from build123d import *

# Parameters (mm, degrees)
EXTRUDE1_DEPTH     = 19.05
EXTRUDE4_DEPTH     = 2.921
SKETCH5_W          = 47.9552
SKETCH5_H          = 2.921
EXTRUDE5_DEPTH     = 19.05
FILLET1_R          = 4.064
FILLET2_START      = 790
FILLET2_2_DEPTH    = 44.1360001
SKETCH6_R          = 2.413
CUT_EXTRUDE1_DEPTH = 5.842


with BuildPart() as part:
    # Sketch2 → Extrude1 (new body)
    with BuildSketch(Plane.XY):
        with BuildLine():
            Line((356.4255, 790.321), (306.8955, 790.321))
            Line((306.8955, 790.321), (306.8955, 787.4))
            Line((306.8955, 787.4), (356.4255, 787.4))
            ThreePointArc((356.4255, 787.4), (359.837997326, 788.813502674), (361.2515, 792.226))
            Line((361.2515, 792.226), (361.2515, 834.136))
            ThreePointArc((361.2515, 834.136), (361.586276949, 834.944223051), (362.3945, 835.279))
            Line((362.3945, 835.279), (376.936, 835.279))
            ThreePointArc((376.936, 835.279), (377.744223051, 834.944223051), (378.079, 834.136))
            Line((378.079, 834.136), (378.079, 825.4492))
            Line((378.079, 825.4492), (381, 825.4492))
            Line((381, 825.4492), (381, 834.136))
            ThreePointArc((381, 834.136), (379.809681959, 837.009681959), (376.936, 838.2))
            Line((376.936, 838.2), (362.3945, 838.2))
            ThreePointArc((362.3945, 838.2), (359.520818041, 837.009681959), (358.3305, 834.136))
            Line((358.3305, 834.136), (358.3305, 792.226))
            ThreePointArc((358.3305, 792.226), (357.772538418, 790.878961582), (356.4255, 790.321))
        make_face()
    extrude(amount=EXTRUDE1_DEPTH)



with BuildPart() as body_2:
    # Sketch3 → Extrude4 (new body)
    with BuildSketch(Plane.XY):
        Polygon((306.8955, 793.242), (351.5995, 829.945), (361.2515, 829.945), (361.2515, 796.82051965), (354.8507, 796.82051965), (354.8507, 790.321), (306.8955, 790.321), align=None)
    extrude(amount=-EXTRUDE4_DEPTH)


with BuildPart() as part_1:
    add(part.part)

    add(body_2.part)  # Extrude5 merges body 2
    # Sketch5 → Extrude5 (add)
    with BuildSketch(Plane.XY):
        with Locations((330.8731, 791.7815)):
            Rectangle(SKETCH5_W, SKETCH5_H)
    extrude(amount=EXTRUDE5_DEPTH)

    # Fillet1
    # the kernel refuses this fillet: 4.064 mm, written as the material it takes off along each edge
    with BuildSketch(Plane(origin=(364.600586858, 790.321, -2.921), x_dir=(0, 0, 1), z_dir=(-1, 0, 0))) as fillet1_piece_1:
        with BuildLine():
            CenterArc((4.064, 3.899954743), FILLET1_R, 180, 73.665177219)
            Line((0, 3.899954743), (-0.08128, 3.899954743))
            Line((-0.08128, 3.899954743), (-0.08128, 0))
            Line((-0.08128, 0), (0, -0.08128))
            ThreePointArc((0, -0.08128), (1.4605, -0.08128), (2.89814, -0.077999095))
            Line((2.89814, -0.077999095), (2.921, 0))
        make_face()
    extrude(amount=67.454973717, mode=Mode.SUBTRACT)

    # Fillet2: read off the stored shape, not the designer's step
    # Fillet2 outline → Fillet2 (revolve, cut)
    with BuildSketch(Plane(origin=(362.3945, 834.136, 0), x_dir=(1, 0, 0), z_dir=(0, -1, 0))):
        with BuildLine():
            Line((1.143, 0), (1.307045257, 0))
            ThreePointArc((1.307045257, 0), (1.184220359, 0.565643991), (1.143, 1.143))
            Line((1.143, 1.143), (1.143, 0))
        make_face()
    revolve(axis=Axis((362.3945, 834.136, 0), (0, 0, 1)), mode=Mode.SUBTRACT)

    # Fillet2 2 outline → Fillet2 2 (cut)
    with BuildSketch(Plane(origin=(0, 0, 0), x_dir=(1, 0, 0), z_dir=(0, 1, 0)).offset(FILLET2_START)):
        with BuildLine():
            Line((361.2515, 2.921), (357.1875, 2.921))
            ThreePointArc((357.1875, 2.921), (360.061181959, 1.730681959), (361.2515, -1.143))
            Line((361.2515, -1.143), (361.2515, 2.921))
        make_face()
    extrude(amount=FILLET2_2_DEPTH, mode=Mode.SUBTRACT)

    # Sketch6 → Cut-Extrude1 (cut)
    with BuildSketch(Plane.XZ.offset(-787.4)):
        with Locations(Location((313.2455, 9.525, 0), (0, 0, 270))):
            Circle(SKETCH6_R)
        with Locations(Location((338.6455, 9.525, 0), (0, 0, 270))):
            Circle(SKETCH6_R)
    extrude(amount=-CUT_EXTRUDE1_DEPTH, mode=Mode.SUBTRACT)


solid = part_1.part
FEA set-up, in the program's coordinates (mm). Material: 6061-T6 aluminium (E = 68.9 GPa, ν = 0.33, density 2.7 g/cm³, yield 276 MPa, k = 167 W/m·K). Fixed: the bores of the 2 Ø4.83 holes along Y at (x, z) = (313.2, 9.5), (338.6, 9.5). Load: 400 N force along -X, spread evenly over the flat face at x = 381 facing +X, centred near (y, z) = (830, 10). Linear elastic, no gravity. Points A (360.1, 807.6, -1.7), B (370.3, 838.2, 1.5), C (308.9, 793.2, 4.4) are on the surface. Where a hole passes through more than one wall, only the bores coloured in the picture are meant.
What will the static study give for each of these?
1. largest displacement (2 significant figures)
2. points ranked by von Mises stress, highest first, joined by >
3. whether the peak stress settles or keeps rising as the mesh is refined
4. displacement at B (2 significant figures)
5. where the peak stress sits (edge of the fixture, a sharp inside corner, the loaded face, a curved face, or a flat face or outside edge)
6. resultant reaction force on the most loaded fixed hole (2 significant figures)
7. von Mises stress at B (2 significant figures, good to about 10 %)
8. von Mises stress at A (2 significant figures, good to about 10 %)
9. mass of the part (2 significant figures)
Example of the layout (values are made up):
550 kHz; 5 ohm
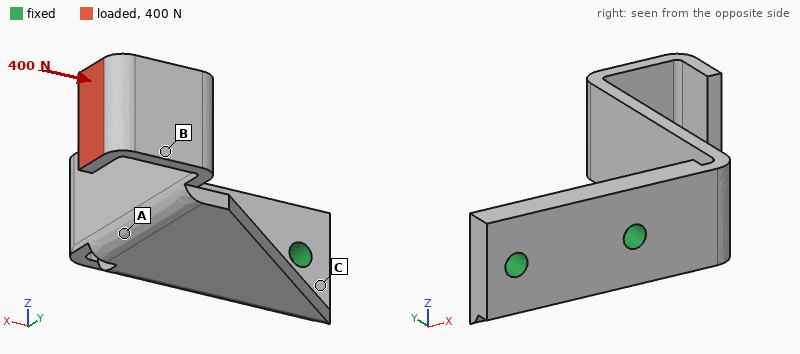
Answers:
0.88 mm; B > A > C; keeps rising; 0.39 mm; a sharp inside corner; 580 N; 97 MPa; 55 MPa; 35 g
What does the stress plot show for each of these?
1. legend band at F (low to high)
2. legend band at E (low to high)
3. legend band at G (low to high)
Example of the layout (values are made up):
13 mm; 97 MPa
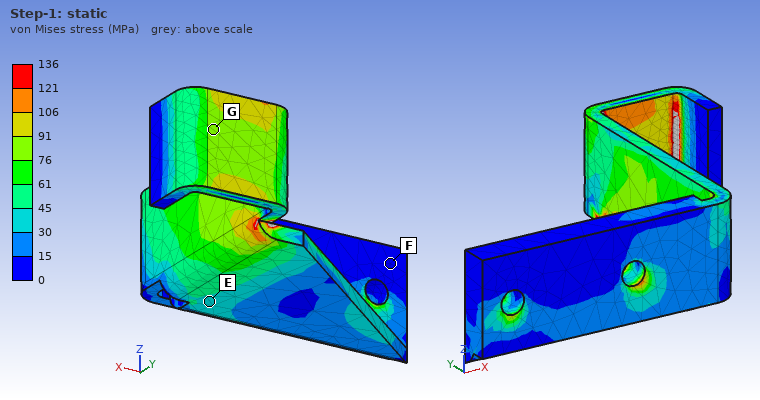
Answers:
0 to 15 MPa; 30 to 45 MPa; 76 to 91 MPa
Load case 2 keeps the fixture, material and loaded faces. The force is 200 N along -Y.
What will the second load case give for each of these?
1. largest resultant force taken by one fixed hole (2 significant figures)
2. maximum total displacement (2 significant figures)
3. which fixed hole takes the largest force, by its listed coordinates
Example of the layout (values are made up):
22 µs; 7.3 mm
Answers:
430 N; 0.75 mm; (338.6, 9.5)
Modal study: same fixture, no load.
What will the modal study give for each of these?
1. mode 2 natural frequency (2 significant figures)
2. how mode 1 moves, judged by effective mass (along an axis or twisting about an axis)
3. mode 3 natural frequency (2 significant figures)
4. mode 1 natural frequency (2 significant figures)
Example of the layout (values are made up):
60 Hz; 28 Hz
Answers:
1700 Hz; along Z; 2300 Hz; 1100 Hz
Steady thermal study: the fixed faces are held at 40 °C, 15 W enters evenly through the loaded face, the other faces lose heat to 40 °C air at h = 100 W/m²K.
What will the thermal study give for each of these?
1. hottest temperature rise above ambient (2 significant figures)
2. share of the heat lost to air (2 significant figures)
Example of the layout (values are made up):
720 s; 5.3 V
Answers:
60 K; 63 %
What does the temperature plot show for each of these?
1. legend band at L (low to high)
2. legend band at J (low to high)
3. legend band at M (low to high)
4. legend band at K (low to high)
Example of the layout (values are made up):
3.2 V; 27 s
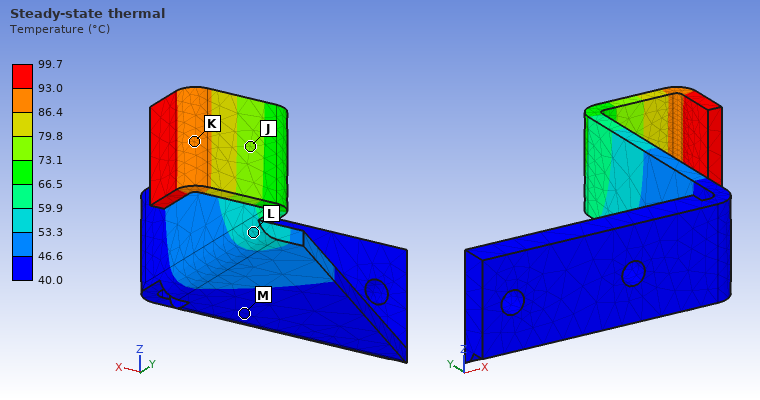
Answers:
53.3 to 59.9 °C; 73.1 to 79.8 °C; 40.0 to 46.6 °C; 86.4 to 93.0 °C
